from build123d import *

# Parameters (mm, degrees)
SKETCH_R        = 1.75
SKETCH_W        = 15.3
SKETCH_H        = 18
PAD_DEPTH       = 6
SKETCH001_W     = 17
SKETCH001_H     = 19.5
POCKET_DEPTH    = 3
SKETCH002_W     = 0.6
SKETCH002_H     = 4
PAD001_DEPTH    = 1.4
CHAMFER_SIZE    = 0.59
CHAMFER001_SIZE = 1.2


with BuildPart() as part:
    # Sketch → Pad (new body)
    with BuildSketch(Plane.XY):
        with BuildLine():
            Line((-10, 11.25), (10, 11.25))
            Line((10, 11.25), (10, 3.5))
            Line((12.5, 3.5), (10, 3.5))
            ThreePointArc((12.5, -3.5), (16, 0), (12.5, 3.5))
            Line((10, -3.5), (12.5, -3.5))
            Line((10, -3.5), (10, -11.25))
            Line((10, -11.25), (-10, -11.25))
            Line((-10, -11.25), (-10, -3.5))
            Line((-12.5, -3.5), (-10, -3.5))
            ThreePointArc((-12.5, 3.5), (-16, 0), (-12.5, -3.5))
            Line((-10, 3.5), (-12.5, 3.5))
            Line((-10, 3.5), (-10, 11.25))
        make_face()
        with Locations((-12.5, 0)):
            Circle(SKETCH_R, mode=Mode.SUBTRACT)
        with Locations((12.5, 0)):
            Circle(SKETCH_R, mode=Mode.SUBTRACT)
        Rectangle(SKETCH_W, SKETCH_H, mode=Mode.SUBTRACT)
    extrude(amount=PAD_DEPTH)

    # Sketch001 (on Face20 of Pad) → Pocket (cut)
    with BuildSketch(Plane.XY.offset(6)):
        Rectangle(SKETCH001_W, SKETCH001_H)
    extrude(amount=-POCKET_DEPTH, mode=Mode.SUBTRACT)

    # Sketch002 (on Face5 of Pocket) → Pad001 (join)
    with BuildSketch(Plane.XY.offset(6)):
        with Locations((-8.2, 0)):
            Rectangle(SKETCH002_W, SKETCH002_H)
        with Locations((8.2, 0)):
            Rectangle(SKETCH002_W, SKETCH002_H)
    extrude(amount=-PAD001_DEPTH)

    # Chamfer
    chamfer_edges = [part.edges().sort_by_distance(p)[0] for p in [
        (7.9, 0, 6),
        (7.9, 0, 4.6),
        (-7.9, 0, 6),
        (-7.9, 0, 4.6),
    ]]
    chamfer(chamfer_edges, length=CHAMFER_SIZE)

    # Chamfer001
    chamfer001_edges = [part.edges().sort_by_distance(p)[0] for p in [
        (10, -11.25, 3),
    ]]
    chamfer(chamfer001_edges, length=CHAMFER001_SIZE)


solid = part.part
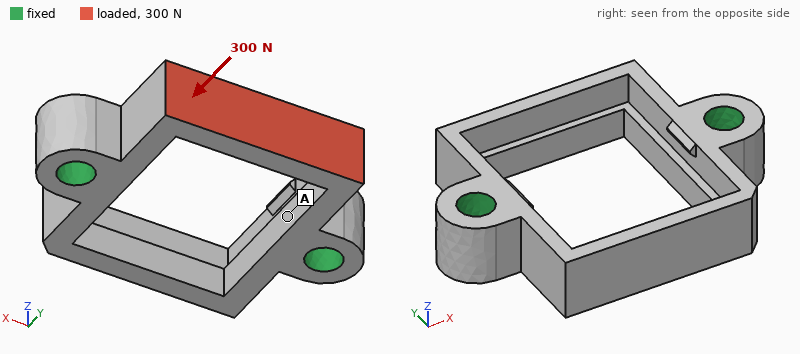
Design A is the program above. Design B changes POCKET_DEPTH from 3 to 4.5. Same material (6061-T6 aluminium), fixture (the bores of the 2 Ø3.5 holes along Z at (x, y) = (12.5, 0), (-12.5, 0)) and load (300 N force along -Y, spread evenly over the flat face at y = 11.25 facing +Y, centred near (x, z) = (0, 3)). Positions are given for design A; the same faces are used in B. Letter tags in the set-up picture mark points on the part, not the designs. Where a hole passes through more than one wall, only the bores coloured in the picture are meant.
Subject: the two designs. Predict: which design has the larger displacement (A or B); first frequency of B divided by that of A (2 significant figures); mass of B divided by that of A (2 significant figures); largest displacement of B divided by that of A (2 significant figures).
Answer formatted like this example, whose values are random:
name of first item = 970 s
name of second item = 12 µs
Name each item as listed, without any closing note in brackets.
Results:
which design has the larger displacement = B
first frequency of B divided by that of A = 0.91
mass of B divided by that of A = 0.93
largest displacement of B divided by that of A = 1.4
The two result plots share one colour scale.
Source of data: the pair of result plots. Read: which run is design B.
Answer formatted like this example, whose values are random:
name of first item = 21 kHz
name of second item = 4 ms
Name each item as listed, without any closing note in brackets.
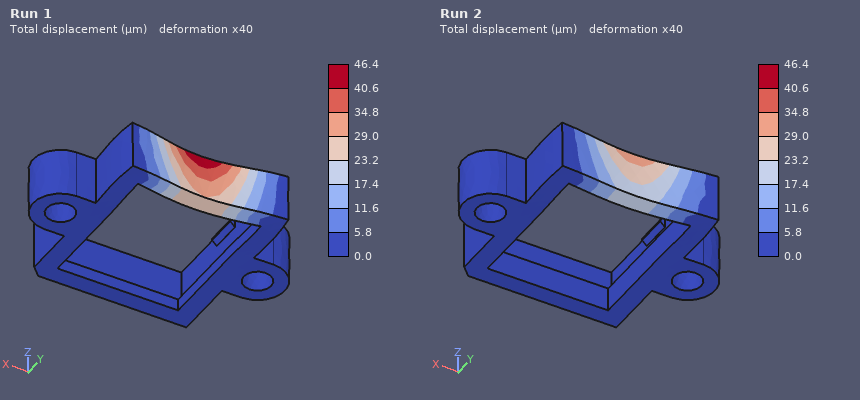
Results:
which run is design B = Run 1
